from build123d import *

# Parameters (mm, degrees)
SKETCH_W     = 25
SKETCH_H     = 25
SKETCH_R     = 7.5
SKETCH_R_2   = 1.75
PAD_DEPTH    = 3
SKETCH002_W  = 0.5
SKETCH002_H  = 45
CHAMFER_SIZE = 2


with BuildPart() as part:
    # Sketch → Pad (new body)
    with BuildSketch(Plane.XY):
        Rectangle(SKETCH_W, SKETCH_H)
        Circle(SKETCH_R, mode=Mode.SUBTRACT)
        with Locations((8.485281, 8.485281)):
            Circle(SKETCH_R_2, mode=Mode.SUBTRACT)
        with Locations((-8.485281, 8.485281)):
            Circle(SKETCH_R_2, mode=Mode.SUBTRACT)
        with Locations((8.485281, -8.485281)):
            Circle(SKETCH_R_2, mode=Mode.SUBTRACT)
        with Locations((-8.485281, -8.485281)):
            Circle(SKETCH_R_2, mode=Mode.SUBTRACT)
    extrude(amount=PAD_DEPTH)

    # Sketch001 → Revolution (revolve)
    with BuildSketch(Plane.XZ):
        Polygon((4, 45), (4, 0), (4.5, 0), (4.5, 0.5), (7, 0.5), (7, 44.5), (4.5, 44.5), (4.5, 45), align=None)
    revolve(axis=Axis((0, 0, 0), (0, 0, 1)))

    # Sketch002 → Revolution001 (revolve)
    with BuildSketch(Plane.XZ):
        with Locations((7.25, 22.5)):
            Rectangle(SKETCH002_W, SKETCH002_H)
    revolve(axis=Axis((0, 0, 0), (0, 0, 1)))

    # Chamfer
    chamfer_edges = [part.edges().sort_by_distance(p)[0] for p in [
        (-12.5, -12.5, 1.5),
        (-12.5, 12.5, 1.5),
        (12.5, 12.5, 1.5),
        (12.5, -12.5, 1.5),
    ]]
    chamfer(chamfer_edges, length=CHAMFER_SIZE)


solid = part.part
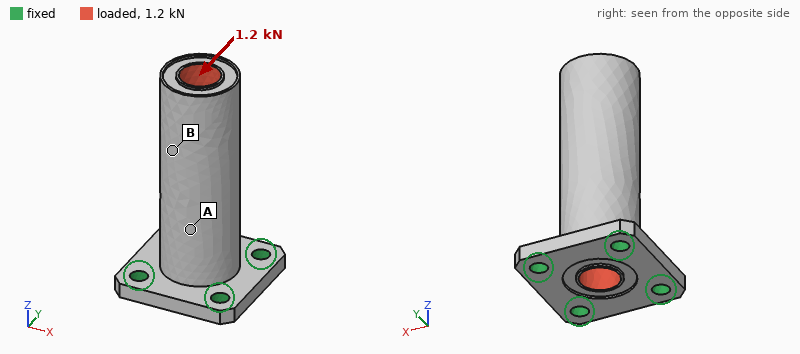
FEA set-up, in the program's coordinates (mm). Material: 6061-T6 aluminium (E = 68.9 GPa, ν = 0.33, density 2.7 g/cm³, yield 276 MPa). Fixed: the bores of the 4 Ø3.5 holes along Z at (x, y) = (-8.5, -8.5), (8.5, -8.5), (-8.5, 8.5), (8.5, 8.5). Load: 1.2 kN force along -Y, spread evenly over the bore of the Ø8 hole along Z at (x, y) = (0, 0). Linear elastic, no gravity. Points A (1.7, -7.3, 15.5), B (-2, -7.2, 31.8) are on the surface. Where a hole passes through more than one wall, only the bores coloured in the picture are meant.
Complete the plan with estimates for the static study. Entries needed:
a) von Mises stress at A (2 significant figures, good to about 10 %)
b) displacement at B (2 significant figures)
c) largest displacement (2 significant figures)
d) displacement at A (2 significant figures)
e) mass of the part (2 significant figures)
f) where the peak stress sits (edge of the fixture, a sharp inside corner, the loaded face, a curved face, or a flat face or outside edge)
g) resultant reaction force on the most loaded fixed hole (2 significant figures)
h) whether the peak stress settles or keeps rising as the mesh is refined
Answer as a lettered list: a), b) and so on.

a) 36 MPa
b) 0.12 mm
c) 0.18 mm
d) 0.053 mm
e) 18 g
f) edge of the fixture
g) 960 N
h) keeps rising
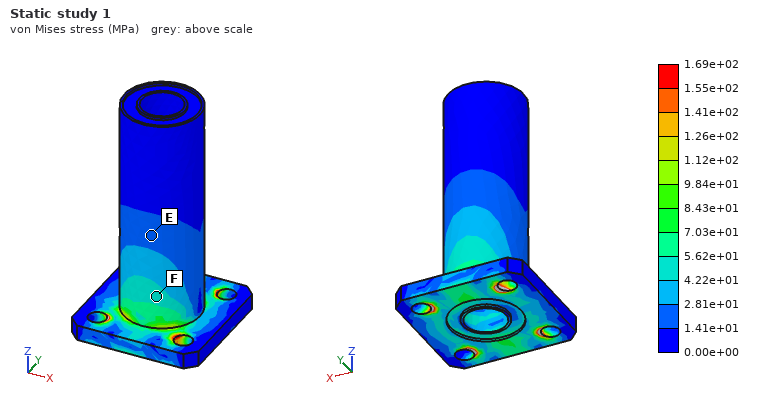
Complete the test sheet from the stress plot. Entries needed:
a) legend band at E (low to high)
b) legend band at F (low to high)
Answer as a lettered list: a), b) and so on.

a) 1.41e+01 to 2.81e+01 MPa
b) 4.22e+01 to 5.62e+01 MPa
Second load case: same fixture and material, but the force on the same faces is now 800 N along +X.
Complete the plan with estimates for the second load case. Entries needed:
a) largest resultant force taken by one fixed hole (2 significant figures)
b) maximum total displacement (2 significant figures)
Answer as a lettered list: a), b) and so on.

a) 640 N
b) 0.12 mm
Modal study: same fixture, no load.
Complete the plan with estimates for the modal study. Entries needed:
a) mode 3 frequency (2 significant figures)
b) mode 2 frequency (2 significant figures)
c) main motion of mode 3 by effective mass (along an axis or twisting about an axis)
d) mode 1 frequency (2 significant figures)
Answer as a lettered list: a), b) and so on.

a) 17 kHz
b) 4200 Hz
c) along Z
d) 4100 Hz
